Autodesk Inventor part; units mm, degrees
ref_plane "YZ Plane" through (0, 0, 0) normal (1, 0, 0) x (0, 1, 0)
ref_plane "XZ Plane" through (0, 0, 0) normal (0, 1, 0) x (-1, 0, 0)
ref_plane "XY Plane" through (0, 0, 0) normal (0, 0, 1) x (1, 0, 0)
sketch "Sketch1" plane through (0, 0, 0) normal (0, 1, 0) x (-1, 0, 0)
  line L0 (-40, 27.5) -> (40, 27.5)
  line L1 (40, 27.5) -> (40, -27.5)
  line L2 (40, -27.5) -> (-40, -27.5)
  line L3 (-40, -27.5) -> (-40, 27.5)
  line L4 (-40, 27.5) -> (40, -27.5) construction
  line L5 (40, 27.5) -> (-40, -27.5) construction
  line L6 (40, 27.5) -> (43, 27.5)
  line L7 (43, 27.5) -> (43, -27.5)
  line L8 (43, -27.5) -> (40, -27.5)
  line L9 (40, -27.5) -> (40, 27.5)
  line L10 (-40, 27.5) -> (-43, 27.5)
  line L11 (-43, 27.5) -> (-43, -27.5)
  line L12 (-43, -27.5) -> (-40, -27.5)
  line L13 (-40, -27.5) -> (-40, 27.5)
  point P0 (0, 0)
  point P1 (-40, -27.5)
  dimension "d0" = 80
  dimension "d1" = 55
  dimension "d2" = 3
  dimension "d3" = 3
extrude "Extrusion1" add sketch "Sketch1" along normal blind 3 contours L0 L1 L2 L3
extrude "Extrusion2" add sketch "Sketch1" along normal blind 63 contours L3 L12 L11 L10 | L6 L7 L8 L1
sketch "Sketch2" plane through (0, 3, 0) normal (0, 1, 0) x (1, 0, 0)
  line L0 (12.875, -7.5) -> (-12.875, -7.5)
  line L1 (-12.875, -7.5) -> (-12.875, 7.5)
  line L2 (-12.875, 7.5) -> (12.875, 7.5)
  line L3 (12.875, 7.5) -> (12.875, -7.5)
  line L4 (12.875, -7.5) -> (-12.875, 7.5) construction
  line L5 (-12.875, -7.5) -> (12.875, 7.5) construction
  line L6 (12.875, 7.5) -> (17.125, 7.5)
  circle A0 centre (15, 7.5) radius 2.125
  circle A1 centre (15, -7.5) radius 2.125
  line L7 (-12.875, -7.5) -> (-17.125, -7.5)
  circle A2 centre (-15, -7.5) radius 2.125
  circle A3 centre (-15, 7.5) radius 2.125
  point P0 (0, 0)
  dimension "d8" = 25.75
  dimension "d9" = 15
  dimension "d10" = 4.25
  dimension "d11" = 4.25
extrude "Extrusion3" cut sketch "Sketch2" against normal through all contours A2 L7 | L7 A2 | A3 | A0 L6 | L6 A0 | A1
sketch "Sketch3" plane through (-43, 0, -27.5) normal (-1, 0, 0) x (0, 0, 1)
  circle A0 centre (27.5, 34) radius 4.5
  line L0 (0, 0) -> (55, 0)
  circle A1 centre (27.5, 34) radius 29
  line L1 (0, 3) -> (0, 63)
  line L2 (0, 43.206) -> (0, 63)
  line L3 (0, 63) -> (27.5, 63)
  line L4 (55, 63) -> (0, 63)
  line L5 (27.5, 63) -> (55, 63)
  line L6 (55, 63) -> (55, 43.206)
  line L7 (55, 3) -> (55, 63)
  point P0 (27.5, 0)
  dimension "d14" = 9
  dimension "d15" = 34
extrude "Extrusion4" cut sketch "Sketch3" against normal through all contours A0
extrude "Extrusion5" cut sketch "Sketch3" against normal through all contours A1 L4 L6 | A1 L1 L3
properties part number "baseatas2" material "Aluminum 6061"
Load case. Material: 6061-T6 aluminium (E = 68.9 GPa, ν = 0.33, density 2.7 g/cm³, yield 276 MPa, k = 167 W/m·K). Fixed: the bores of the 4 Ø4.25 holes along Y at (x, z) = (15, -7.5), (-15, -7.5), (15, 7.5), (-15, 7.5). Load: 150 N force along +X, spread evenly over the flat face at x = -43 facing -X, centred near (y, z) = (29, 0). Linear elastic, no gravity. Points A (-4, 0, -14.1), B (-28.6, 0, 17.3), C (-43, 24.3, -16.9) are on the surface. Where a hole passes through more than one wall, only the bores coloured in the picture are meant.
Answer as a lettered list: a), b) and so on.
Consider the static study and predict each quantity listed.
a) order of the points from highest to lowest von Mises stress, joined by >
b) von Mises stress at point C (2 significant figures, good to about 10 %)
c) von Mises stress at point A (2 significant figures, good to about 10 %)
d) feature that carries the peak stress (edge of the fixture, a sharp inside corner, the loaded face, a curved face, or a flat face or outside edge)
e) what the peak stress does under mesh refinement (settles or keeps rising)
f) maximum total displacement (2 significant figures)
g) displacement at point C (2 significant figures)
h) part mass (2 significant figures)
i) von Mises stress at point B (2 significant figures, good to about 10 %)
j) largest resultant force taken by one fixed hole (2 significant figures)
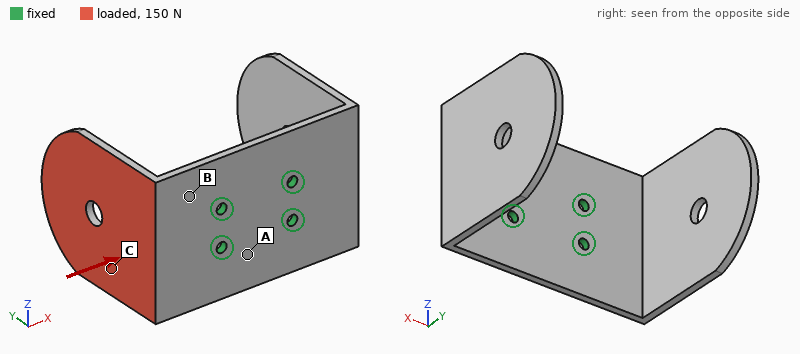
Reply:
a) B > C > A
b) 18 MPa
c) 6.3 MPa
d) edge of the fixture
e) keeps rising
f) 1.2 mm
g) 0.41 mm
h) 86 g
i) 43 MPa
j) 67 N
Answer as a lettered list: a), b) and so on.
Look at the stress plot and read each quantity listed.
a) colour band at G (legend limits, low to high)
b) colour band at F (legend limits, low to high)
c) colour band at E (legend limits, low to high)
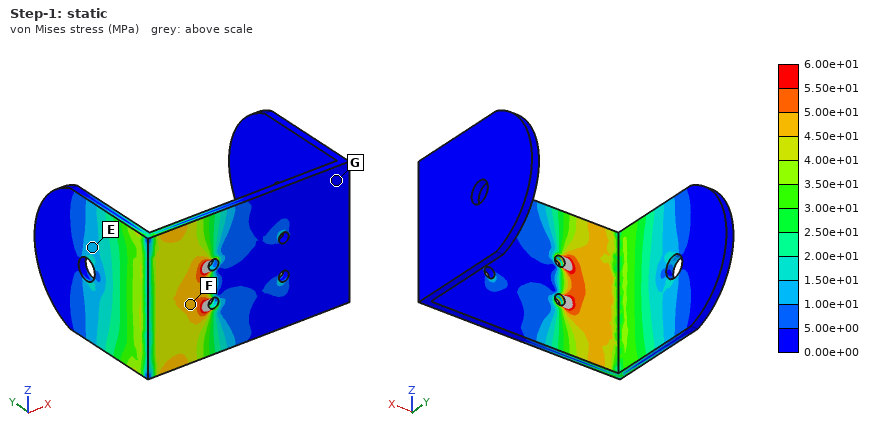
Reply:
a) 0.00e+00 to 5.00e+00 MPa
b) 4.50e+01 to 5.00e+01 MPa
c) 1.00e+01 to 1.50e+01 MPa
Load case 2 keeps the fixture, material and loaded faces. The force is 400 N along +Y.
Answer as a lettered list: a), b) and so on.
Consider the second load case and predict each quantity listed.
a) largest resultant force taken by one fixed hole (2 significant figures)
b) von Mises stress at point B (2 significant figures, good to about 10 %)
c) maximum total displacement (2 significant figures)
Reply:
a) 250 N
b) 62 MPa
c) 1.2 mm
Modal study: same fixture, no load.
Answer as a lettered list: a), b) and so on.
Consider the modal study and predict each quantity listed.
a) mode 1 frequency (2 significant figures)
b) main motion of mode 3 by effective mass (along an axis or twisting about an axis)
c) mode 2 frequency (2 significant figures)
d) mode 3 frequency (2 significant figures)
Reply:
a) 440 Hz
b) twisting about Y
c) 450 Hz
d) 790 Hz
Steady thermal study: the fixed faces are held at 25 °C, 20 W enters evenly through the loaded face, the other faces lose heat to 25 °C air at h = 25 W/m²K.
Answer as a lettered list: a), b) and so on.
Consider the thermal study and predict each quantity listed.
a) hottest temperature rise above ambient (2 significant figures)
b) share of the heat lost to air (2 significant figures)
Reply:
a) 36 K
b) 18 %
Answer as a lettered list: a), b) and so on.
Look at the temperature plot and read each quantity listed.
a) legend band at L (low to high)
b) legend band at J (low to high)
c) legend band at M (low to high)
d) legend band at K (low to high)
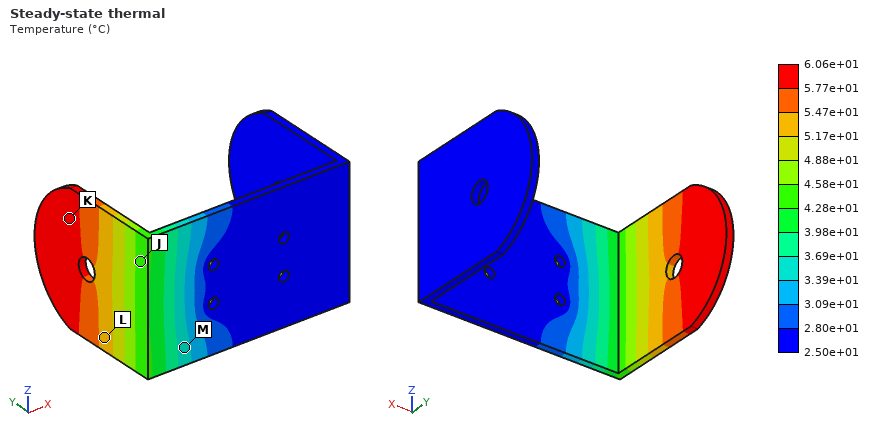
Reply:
a) 5.17e+01 to 5.47e+01 °C
b) 4.28e+01 to 4.58e+01 °C
c) 3.39e+01 to 3.69e+01 °C
d) 5.77e+01 to 6.06e+01 °C
